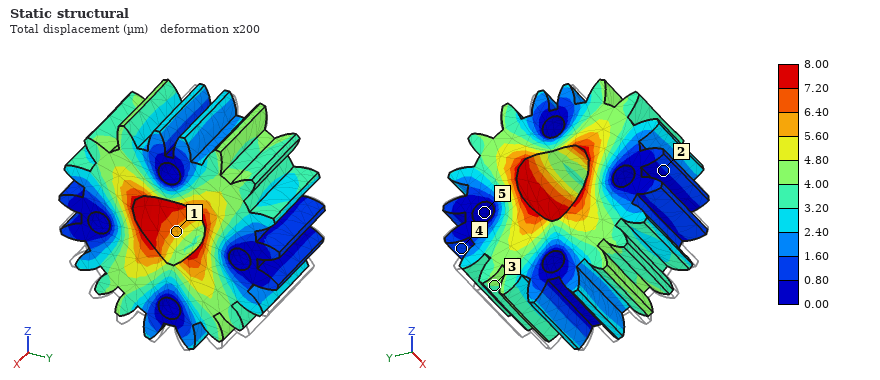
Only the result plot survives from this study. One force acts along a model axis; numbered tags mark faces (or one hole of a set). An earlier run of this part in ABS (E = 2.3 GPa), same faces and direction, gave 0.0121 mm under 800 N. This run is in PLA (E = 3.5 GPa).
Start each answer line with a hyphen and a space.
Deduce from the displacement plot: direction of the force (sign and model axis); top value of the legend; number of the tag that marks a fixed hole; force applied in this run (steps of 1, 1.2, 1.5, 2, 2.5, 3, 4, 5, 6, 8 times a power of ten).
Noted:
- +Z
- 8.00 µm
- 5
- 800 N
